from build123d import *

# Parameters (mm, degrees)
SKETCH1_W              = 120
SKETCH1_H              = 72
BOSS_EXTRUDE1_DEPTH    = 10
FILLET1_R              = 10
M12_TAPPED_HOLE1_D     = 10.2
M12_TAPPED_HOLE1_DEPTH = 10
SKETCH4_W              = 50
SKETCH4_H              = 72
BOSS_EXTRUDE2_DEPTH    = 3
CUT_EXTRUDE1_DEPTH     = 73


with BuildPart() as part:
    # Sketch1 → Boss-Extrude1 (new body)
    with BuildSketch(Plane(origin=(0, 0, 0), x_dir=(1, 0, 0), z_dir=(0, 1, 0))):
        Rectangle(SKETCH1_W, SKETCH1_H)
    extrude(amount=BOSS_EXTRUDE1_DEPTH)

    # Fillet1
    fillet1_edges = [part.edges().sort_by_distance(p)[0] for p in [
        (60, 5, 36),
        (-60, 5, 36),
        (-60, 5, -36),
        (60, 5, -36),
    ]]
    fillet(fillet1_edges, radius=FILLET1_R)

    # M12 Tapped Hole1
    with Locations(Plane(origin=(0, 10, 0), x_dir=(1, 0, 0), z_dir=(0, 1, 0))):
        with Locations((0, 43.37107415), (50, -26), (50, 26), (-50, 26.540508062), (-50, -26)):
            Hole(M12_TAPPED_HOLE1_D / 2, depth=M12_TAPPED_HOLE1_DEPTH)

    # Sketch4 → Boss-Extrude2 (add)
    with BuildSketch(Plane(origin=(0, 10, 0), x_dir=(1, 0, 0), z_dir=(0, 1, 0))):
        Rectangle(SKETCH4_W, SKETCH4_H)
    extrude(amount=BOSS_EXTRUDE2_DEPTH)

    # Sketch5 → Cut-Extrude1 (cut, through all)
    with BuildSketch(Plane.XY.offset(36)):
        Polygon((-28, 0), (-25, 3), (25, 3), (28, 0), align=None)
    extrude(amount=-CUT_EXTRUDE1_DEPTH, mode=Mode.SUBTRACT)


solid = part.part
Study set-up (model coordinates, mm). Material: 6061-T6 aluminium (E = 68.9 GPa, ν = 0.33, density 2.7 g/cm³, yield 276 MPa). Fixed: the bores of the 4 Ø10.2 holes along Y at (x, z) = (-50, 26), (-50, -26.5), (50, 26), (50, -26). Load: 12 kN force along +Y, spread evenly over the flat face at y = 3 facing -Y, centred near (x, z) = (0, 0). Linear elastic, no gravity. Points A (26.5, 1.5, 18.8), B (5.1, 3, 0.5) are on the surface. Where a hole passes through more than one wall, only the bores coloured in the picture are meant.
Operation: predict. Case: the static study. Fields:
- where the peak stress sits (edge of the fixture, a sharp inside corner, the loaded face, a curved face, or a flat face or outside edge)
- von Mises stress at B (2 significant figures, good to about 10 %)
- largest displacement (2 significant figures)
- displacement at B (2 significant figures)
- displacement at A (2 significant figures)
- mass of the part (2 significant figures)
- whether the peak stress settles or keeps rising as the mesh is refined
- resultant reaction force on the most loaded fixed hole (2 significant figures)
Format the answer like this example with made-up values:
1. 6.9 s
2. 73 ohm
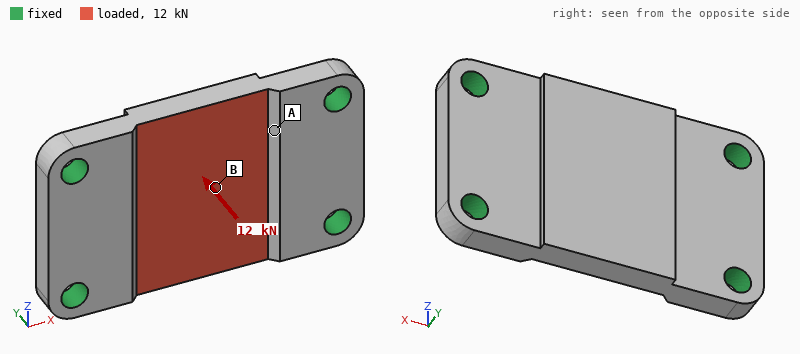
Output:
1. edge of the fixture
2. 39 MPa
3. 0.12 mm
4. 0.11 mm
5. 0.061 mm
6. 220 g
7. keeps rising
8. 4.9 kN
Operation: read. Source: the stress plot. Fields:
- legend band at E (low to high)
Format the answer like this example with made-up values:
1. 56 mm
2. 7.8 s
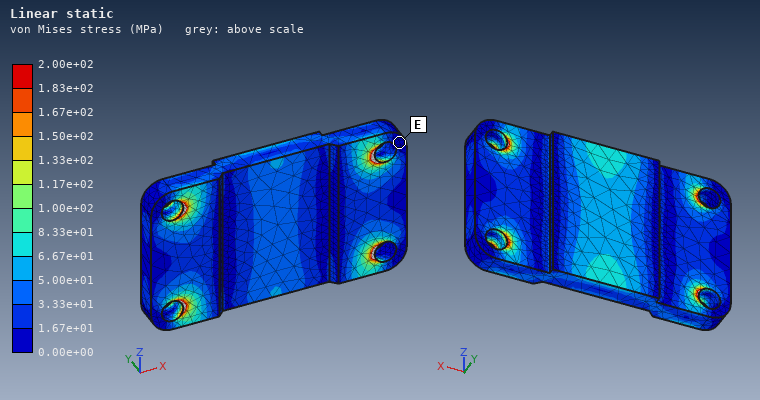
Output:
1. 0.00e+00 to 1.67e+01 MPa
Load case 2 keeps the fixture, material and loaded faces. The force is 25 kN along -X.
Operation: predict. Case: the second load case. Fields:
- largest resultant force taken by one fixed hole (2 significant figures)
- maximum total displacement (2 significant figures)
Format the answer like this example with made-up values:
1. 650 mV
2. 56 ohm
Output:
1. 6.4 kN
2. 19 µm
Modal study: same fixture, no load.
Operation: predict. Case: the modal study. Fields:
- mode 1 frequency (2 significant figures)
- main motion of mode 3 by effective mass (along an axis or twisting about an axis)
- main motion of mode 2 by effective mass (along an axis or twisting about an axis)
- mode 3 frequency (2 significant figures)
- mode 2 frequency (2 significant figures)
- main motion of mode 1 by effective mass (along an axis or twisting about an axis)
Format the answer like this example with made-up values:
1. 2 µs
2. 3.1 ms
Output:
1. 5300 Hz
2. twisting about Z
3. twisting about X
4. 12 kHz
5. 7100 Hz
6. along Y
